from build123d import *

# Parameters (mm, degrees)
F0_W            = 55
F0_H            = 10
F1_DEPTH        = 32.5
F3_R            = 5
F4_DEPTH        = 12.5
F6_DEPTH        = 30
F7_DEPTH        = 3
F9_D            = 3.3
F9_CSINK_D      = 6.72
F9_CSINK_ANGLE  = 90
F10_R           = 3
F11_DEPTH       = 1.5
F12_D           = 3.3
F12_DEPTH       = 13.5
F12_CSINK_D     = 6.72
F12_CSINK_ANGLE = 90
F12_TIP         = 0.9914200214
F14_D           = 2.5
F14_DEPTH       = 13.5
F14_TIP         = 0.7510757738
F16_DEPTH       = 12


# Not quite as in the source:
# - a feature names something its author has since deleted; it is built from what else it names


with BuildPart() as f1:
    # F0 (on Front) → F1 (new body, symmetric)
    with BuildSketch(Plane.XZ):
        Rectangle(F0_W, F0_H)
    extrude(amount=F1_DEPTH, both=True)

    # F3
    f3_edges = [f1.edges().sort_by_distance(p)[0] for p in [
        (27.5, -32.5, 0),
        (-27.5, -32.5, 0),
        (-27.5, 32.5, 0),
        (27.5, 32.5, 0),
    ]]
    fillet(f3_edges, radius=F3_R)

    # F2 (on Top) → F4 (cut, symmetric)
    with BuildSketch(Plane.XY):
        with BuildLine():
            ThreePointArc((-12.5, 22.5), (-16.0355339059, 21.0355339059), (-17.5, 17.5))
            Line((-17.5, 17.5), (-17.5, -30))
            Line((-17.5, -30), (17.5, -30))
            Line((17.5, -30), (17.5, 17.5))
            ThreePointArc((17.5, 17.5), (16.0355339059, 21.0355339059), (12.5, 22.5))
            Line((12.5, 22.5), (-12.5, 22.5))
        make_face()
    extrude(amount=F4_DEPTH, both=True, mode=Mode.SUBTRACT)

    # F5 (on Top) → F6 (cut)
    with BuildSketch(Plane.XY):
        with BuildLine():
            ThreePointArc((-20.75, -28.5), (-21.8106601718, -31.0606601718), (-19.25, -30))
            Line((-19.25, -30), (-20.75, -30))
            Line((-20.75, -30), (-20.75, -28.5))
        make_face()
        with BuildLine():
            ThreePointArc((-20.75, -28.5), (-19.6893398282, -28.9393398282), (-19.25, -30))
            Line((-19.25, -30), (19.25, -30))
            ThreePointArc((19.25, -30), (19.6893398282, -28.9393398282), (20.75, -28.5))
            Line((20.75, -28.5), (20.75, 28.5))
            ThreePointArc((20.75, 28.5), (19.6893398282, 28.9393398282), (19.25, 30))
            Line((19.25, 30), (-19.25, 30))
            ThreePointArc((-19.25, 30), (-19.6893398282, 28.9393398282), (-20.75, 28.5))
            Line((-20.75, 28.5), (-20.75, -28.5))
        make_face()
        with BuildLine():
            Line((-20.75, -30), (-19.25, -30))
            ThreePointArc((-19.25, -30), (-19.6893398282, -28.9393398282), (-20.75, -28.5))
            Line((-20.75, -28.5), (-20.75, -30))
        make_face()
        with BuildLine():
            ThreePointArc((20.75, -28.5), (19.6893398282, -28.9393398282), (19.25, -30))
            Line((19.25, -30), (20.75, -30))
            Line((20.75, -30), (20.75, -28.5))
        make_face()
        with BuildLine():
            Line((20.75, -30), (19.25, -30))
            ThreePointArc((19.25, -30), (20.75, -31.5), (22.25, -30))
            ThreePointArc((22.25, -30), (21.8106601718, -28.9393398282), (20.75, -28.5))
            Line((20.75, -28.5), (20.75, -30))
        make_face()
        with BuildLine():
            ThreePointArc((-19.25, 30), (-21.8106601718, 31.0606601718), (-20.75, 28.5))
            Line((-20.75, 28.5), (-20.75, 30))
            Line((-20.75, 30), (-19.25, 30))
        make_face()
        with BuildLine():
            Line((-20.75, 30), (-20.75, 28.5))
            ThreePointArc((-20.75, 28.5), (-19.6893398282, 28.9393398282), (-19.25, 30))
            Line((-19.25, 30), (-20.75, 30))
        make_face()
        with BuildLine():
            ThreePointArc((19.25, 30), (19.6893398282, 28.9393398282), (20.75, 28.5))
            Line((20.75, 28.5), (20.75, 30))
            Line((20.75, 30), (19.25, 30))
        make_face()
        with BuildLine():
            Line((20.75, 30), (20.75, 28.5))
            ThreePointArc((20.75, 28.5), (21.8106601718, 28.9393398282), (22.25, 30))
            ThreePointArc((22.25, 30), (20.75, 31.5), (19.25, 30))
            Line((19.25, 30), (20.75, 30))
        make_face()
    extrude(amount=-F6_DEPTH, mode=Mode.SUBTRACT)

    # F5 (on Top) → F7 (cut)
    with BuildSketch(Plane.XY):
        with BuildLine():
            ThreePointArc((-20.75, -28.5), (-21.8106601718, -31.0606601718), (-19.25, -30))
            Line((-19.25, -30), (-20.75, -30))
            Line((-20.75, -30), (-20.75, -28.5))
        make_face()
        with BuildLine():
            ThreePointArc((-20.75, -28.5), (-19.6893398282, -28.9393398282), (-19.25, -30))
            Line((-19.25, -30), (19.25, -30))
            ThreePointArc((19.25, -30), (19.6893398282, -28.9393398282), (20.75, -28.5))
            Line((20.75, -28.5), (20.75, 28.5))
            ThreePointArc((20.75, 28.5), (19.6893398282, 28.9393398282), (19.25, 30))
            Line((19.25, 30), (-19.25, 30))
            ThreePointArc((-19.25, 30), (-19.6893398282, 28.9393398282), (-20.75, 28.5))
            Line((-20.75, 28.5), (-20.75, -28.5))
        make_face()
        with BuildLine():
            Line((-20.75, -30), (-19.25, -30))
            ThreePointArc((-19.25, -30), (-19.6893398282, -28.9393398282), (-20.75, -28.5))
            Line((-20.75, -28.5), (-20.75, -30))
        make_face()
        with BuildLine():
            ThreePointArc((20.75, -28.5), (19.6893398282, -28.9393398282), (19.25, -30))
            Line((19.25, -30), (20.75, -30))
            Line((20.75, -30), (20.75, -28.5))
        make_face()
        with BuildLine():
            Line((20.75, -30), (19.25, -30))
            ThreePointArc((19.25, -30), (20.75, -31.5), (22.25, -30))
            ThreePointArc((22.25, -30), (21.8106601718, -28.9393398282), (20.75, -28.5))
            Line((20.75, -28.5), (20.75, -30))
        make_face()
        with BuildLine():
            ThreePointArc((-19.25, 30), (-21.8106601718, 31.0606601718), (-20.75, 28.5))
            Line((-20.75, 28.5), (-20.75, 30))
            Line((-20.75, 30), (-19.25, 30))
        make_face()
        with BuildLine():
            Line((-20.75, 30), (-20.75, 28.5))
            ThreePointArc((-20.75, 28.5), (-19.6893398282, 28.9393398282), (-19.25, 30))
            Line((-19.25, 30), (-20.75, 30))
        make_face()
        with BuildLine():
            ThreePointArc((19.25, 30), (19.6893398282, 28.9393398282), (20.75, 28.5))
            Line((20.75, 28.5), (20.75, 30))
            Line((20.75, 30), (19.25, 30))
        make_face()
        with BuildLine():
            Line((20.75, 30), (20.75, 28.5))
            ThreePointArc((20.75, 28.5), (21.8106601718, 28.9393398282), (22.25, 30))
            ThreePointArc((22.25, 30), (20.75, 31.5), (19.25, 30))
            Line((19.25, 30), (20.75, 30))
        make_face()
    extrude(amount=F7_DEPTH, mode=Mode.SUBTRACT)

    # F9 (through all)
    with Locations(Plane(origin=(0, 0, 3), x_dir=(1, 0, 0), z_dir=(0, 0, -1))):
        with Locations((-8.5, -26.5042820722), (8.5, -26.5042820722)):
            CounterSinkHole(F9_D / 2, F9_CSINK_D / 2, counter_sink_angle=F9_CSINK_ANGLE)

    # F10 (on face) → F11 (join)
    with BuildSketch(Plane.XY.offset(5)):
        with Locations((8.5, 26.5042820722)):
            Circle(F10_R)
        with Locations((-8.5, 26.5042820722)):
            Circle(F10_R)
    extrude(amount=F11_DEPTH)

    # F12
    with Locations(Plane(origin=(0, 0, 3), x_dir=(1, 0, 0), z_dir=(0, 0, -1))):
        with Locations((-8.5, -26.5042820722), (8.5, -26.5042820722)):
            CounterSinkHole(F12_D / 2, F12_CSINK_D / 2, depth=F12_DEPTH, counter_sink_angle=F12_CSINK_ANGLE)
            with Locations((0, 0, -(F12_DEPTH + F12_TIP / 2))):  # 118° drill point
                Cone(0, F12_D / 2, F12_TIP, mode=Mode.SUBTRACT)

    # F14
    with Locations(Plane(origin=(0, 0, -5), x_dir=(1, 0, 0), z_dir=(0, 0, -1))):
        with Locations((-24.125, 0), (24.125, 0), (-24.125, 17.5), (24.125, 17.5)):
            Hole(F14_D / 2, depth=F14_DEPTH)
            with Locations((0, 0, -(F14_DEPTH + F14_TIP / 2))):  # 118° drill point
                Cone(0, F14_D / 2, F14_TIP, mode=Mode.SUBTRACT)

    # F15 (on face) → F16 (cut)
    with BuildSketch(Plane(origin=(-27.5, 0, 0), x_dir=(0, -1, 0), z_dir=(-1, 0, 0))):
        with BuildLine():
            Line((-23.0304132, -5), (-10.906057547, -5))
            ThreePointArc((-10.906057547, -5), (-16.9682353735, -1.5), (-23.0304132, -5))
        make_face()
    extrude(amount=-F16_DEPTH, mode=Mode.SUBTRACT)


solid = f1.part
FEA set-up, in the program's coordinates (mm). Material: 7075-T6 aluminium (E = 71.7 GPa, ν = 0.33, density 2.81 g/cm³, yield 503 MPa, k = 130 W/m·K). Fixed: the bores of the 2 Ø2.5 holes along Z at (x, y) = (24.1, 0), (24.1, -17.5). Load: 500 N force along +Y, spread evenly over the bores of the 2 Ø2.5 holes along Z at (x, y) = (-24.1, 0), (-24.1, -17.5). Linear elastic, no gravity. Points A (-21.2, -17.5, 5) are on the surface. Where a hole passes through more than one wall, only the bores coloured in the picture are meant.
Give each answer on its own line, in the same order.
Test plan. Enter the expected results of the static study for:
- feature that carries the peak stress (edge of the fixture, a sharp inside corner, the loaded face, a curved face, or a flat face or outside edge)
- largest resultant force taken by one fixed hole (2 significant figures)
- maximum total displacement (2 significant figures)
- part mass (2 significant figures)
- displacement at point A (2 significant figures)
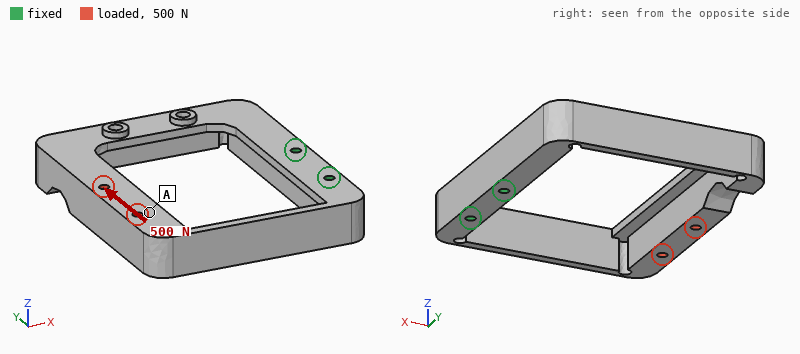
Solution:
a flat face or outside edge
840 N
0.90 mm
32 g
0.72 mm
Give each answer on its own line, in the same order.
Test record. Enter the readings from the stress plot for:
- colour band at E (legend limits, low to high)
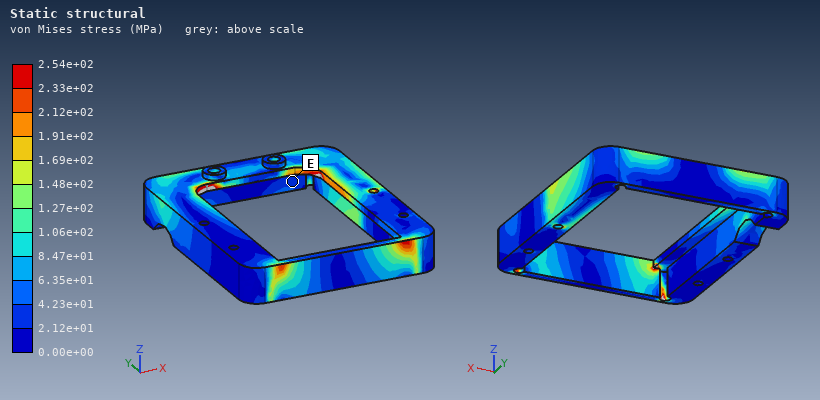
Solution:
2.12e+01 to 4.23e+01 MPa
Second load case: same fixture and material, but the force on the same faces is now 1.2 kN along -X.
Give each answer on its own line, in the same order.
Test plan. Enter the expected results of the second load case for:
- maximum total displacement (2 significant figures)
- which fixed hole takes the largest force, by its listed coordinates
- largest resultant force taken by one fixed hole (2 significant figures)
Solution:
0.36 mm
(24.1, -17.5)
720 N
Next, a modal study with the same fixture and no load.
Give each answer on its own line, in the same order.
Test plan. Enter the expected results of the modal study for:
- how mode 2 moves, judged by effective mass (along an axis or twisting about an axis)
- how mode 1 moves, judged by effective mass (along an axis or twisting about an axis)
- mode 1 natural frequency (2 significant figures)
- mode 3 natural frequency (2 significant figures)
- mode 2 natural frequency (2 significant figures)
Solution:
along Y
along Z
780 Hz
1800 Hz
1000 Hz
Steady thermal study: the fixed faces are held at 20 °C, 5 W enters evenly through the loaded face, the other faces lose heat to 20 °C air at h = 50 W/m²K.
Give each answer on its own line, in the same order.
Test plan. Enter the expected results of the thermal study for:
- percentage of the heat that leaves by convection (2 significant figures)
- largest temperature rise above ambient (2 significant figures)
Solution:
66 %
20 K
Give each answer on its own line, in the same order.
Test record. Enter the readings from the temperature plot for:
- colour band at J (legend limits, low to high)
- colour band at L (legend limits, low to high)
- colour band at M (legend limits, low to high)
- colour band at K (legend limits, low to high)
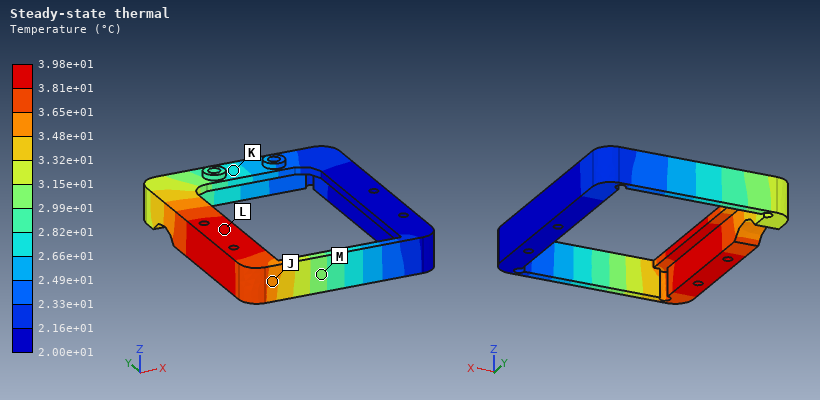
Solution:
3.48e+01 to 3.65e+01 °C
3.81e+01 to 3.98e+01 °C
2.99e+01 to 3.15e+01 °C
2.66e+01 to 2.82e+01 °C
